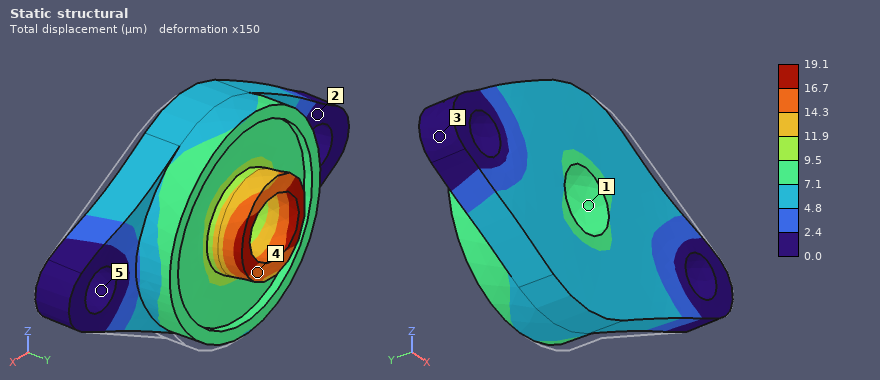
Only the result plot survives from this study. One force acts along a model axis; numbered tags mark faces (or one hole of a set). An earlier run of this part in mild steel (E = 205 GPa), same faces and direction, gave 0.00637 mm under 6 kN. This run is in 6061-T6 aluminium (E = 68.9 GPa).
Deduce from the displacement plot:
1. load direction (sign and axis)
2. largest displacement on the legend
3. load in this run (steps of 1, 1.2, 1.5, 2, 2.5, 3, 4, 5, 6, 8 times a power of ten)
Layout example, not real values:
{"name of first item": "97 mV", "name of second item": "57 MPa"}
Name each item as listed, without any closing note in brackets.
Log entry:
{"load direction": "-X", "largest displacement on the legend": "19.1 µm", "load in this run": "6 kN"}
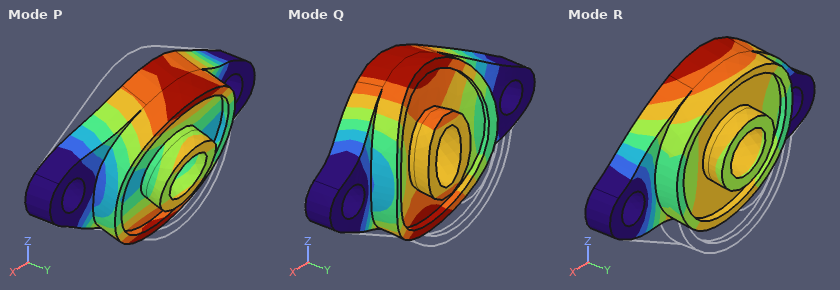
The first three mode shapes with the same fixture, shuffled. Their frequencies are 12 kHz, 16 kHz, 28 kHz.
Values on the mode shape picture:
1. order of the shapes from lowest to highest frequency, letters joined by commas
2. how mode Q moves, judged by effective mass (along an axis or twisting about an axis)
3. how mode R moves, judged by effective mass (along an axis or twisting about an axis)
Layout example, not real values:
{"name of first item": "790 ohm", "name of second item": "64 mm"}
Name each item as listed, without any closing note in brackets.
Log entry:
{"order of the shapes from lowest to highest frequency, letters joined by commas": "P, Q, R", "how mode Q moves, judged by effective mass": "along Y", "how mode R moves, judged by effective mass": "along Z"}
